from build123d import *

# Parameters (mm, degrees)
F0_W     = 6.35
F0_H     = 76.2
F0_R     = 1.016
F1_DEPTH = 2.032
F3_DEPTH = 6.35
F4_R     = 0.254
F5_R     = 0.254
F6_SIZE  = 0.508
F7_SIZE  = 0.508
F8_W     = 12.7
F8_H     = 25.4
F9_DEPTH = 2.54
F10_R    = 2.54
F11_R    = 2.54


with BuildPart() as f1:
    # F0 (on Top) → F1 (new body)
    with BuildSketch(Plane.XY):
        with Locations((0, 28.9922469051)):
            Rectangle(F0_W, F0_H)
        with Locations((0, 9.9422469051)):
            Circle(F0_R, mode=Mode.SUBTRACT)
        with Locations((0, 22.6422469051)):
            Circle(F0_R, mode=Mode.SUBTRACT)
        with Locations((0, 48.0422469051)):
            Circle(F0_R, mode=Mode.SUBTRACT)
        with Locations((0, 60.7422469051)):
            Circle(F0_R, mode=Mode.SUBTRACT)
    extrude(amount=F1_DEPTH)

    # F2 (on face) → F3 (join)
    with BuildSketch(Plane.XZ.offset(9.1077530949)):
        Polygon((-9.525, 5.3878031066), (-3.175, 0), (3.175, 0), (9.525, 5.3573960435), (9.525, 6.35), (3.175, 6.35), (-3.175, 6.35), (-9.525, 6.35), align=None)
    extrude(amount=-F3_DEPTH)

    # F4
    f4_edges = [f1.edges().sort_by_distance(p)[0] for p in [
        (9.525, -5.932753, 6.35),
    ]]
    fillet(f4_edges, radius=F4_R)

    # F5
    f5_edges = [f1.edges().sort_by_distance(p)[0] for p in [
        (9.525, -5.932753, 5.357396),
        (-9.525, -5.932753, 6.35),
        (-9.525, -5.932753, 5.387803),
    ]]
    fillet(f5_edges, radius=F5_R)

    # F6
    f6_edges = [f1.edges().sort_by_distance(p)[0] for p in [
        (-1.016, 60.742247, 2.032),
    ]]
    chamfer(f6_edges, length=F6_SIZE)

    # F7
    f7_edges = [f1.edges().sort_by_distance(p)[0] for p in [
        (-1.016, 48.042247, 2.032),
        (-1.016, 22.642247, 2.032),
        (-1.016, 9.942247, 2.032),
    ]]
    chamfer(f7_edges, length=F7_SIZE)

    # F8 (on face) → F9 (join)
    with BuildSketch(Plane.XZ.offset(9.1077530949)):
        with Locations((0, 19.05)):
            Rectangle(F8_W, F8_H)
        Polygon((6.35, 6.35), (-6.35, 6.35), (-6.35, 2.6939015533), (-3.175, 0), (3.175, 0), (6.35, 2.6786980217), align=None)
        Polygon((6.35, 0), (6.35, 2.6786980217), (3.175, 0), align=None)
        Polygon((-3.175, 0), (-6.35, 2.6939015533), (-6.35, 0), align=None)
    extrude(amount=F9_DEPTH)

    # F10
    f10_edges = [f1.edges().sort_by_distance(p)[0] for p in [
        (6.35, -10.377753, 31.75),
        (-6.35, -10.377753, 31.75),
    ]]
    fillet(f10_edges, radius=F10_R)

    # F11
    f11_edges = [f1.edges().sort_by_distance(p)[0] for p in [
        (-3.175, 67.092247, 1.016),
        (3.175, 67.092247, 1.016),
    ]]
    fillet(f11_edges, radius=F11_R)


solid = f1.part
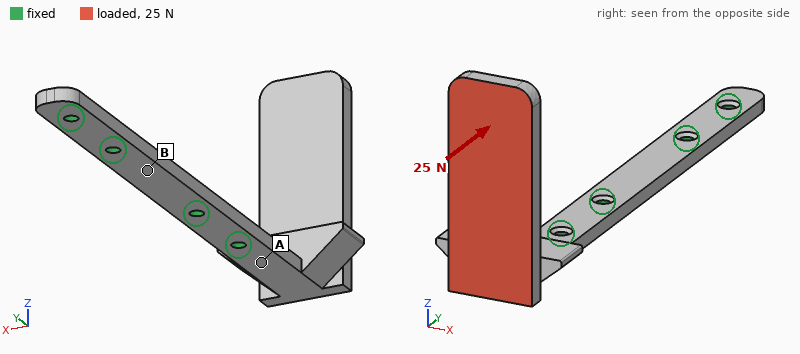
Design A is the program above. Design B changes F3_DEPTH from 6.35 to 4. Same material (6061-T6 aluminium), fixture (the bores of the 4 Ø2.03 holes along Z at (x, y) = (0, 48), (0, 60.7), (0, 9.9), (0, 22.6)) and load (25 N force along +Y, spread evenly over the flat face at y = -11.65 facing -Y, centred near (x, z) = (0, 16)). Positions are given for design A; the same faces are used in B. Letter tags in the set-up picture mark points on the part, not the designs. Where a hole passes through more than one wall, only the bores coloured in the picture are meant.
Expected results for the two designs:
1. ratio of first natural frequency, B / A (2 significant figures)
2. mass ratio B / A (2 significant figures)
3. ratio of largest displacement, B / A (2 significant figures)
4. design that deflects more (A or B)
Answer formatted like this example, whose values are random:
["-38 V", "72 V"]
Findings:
["0.97", "0.93", "1.1", "B"]
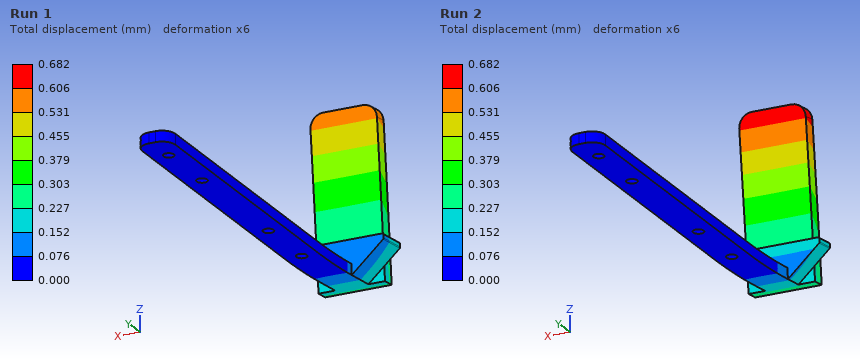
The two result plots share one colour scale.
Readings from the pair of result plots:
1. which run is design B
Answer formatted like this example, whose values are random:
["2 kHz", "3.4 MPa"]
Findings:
["Run 2"]
